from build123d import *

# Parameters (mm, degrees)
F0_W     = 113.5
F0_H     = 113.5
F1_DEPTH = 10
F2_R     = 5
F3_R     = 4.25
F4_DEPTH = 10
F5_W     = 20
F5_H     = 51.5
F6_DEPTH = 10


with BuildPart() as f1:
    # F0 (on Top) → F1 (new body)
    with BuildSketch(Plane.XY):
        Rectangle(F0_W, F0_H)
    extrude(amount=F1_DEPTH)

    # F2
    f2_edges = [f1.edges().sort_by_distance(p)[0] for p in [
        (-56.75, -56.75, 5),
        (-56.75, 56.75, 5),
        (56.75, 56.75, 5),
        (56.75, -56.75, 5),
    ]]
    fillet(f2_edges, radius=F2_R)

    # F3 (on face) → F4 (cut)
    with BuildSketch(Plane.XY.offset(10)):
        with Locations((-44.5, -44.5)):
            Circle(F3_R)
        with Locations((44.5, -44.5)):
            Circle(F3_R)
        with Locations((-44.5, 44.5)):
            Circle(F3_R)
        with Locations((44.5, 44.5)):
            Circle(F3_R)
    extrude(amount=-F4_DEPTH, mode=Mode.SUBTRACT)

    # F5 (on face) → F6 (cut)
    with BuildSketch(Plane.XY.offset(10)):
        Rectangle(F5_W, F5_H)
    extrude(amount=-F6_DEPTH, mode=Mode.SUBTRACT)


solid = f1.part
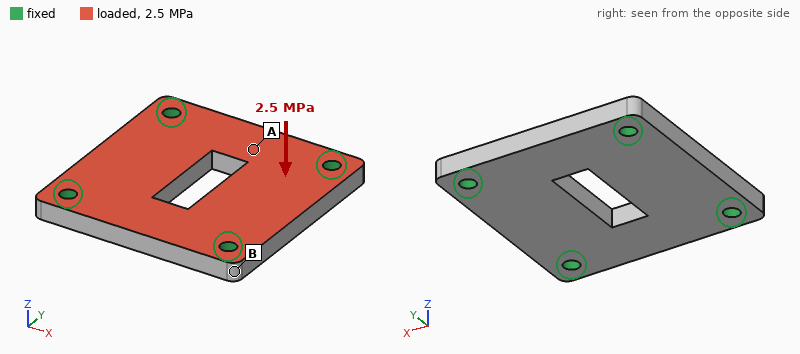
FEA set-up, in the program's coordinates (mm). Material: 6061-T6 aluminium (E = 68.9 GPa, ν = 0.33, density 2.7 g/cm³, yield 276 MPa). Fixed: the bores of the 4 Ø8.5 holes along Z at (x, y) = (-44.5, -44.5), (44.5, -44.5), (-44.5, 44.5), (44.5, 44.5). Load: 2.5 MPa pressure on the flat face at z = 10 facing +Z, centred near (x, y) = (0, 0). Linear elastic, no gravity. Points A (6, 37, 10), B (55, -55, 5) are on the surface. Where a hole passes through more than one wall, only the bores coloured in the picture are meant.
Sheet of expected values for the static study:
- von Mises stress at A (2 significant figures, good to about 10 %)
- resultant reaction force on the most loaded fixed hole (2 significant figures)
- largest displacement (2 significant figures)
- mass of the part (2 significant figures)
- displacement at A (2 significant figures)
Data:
60 MPa
7.3 kN
0.21 mm
310 g
0.12 mm
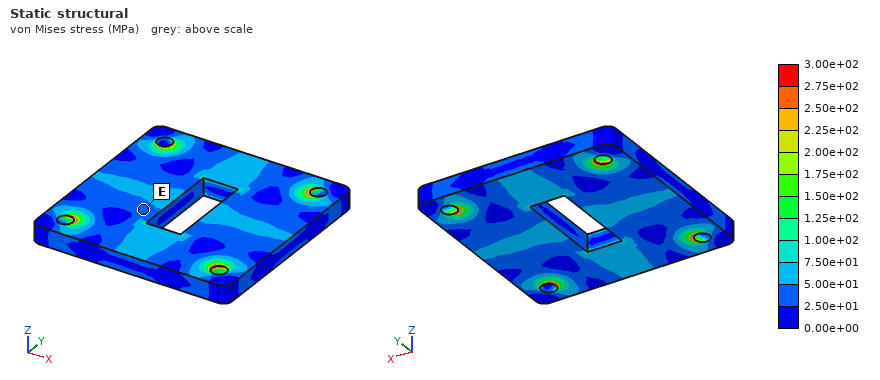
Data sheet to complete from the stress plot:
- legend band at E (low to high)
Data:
2.50e+01 to 5.00e+01 MPa
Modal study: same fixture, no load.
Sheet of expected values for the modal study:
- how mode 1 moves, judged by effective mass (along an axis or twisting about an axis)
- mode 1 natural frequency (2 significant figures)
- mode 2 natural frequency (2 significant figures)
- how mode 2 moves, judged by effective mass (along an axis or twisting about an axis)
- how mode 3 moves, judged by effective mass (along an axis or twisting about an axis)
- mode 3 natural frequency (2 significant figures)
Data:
along Z
4400 Hz
6300 Hz
twisting about Y
twisting about X
6900 Hz
